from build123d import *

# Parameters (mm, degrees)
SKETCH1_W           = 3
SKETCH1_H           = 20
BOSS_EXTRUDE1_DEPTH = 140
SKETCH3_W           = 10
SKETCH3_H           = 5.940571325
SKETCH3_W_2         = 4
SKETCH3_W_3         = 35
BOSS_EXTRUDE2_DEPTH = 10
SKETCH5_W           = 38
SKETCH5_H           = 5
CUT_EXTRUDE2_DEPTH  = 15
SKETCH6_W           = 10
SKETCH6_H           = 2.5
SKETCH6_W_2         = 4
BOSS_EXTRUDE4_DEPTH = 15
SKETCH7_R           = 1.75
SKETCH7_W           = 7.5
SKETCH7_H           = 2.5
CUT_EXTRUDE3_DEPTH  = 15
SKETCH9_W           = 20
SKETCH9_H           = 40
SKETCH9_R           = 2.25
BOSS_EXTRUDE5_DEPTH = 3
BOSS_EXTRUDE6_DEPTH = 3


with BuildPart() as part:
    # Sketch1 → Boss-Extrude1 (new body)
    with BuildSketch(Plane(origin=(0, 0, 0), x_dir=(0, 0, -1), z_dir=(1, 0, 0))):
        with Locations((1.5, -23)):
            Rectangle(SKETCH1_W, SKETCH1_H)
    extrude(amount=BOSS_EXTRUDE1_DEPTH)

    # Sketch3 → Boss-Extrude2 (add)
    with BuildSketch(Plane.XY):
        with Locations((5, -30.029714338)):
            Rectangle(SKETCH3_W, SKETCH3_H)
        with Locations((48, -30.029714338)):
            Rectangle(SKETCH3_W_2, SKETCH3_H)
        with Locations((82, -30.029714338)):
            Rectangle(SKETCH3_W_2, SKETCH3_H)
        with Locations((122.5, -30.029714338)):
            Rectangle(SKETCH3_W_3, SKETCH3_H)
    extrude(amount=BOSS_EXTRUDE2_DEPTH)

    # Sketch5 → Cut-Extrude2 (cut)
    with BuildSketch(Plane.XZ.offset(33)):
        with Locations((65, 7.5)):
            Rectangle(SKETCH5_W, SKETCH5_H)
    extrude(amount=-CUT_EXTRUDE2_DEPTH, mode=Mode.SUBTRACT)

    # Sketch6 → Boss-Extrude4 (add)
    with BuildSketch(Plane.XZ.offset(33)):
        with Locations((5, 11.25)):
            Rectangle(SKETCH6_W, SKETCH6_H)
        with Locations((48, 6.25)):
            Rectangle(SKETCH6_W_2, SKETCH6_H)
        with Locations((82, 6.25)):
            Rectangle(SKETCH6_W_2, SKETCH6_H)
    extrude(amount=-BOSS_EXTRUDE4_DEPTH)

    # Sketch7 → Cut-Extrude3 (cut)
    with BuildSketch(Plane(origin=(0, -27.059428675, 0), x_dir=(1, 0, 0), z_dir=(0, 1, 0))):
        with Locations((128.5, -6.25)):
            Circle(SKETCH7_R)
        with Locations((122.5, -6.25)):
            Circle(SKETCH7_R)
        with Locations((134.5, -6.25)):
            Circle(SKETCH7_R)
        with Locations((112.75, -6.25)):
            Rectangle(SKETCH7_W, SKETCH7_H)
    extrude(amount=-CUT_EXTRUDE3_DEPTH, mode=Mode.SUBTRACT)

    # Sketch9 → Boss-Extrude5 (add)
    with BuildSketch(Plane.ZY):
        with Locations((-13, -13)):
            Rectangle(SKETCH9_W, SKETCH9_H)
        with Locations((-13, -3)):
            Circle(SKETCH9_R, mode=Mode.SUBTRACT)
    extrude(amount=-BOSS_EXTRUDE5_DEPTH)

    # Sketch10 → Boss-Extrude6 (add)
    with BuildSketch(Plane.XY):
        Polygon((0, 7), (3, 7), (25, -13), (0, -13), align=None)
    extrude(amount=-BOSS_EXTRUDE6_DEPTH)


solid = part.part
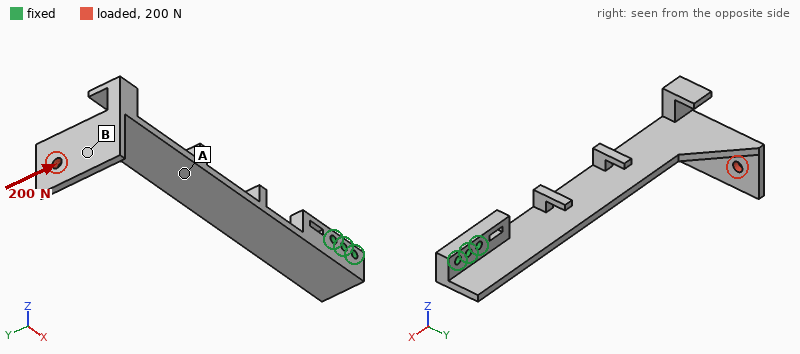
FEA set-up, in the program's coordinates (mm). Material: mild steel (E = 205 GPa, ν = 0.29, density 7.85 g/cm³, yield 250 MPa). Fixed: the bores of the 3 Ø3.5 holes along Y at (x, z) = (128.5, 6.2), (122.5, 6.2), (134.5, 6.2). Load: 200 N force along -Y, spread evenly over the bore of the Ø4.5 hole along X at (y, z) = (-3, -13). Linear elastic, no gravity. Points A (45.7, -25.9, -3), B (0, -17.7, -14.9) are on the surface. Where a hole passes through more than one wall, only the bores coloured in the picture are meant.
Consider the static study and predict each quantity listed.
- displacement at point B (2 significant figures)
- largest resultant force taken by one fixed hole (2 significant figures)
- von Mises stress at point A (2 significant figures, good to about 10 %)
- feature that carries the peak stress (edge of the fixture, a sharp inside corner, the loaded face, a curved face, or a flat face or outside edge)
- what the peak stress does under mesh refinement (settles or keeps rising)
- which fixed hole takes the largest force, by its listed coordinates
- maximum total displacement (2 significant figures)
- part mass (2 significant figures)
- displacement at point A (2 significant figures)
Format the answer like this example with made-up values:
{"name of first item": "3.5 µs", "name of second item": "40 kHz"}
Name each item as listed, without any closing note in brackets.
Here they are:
{"displacement at point B": "0.71 mm", "largest resultant force taken by one fixed hole": "1.3 kN", "von Mises stress at point A": "75 MPa", "feature that carries the peak stress": "edge of the fixture", "what the peak stress does under mesh refinement": "keeps rising", "which fixed hole takes the largest force, by its listed coordinates": "(122.5, 6.2)", "maximum total displacement": "1.1 mm", "part mass": "120 g", "displacement at point A": "0.24 mm"}
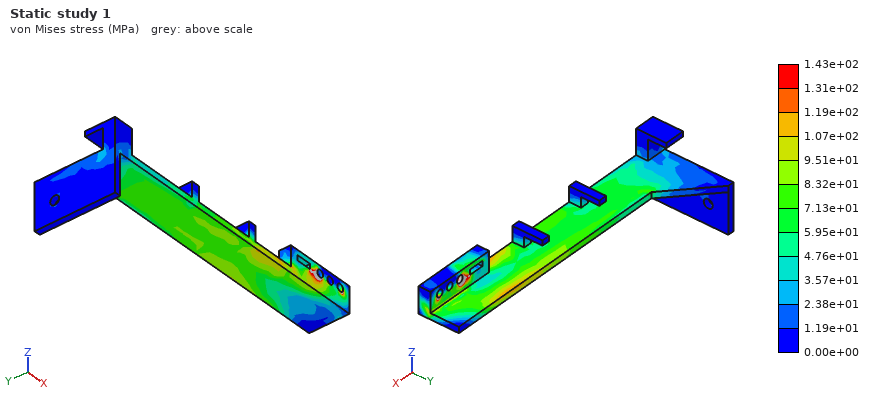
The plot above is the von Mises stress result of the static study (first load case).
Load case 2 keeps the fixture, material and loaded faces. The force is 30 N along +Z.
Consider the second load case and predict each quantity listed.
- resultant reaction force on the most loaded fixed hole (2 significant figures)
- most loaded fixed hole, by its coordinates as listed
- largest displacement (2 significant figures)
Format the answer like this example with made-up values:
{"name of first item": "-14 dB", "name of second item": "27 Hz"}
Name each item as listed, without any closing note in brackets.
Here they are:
{"resultant reaction force on the most loaded fixed hole": "340 N", "most loaded fixed hole, by its coordinates as listed": "(122.5, 6.2)", "largest displacement": "1.6 mm"}
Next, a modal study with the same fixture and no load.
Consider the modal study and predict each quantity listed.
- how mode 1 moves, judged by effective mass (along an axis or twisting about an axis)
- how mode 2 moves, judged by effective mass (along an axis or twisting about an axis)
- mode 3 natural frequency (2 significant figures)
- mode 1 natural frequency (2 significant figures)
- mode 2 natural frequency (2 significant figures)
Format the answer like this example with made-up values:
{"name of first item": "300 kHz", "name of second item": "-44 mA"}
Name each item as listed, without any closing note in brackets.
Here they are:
{"how mode 1 moves, judged by effective mass": "along Z", "how mode 2 moves, judged by effective mass": "along Y", "mode 3 natural frequency": "640 Hz", "mode 1 natural frequency": "110 Hz", "mode 2 natural frequency": "480 Hz"}
